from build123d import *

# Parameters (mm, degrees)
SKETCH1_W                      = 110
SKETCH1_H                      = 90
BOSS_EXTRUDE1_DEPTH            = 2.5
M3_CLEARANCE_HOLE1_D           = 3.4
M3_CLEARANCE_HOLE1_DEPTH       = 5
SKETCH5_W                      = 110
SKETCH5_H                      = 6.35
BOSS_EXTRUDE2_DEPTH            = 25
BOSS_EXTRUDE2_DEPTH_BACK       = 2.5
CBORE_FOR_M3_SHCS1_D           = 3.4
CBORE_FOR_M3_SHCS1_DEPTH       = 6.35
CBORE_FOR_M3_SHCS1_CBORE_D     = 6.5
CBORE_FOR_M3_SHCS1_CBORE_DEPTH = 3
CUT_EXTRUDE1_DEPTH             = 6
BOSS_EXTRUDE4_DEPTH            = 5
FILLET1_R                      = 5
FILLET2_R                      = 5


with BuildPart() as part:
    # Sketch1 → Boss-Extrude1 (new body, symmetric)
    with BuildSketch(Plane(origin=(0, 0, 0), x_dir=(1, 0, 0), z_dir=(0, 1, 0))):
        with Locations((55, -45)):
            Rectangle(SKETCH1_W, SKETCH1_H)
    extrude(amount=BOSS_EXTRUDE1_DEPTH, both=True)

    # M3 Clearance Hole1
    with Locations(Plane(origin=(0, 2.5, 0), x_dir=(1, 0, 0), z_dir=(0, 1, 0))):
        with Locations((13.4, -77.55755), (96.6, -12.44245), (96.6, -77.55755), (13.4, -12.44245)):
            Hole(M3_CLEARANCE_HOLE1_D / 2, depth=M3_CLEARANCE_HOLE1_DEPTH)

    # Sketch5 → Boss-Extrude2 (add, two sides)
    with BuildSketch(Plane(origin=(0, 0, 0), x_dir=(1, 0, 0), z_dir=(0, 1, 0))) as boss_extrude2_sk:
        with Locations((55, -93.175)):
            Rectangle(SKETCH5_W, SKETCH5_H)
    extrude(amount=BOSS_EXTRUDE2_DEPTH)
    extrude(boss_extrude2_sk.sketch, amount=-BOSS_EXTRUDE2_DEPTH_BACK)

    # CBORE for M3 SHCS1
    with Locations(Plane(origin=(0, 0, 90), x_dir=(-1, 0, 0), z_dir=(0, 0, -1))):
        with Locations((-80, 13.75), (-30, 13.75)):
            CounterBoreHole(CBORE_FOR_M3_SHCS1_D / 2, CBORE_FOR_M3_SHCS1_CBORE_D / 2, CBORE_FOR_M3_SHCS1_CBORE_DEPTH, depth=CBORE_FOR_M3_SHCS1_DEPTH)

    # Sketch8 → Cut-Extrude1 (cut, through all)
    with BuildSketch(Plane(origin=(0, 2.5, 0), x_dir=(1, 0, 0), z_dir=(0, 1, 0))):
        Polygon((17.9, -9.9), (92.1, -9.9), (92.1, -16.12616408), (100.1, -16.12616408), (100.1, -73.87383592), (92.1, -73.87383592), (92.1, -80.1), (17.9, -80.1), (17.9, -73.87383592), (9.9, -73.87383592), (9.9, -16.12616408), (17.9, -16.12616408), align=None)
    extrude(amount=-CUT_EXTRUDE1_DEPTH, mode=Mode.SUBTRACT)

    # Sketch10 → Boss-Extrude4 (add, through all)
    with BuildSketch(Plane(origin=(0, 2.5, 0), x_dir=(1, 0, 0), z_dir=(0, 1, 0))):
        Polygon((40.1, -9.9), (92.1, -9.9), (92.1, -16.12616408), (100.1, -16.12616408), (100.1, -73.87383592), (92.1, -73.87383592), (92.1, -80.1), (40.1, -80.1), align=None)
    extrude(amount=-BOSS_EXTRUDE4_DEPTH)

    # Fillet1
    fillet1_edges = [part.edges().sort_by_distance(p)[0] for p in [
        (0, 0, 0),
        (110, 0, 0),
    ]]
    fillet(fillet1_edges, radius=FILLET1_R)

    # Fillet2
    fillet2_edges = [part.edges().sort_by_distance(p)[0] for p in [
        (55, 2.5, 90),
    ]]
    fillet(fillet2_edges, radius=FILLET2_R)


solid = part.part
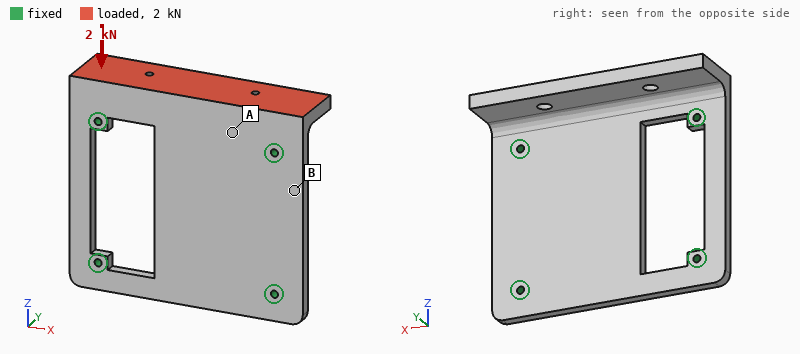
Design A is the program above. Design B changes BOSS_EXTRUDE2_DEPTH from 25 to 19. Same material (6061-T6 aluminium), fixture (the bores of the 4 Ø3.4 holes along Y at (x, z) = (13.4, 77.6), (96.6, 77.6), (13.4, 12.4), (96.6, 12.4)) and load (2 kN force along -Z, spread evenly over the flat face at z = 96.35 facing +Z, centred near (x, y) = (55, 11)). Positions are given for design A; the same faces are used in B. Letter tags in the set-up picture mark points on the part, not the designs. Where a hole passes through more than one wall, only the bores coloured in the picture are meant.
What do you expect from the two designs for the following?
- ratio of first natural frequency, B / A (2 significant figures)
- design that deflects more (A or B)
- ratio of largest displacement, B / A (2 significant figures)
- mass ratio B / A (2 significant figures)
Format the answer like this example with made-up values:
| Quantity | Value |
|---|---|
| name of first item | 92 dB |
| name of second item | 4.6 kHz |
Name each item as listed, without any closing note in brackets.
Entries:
| Quantity | Value |
|---|---|
| ratio of first natural frequency, B / A | 1.1 |
| design that deflects more | A |
| ratio of largest displacement, B / A | 0.61 |
| mass ratio B / A | 0.93 |
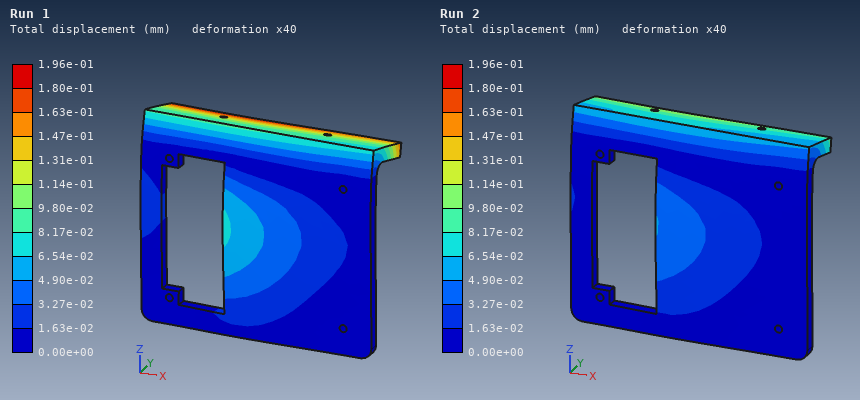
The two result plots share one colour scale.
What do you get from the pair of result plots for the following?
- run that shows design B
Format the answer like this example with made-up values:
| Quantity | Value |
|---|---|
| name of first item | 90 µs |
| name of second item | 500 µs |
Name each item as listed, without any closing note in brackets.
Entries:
| Quantity | Value |
|---|---|
| run that shows design B | Run 2 |
